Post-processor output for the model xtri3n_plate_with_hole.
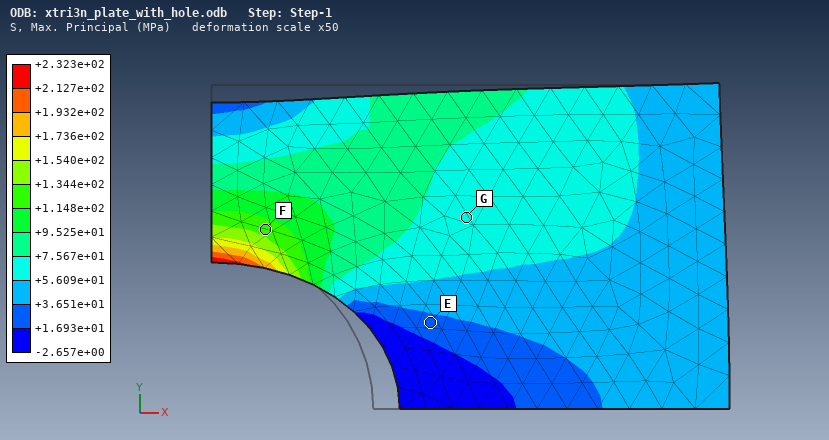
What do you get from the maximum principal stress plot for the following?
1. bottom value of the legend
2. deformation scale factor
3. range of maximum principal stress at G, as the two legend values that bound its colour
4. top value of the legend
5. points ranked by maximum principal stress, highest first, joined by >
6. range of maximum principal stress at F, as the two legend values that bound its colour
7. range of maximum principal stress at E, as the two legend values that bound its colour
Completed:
-2.657e+00 MPa
50
+5.609e+01 to +7.567e+01 MPa
+2.323e+02 MPa
F > G > E
+1.148e+02 to +1.344e+02 MPa
+1.693e+01 to +3.651e+01 MPa
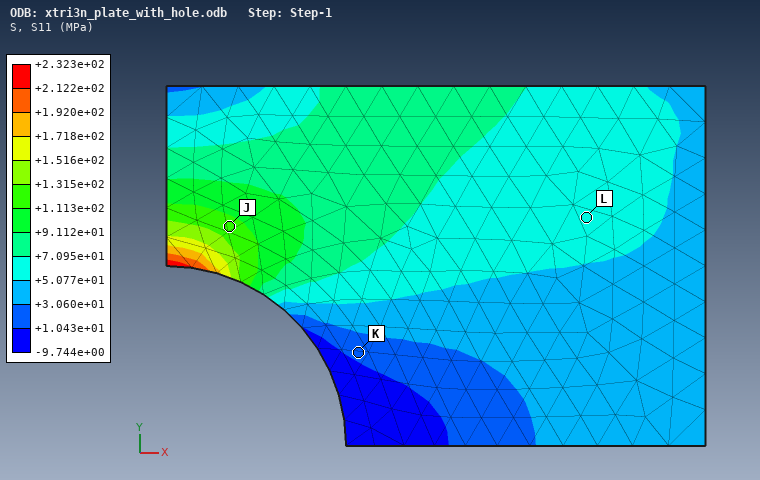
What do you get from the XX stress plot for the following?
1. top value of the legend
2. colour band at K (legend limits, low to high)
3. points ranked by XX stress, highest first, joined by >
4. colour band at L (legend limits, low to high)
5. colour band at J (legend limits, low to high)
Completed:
+2.323e+02 MPa
+1.043e+01 to +3.060e+01 MPa
J > L > K
+5.077e+01 to +7.095e+01 MPa
+1.113e+02 to +1.315e+02 MPa
